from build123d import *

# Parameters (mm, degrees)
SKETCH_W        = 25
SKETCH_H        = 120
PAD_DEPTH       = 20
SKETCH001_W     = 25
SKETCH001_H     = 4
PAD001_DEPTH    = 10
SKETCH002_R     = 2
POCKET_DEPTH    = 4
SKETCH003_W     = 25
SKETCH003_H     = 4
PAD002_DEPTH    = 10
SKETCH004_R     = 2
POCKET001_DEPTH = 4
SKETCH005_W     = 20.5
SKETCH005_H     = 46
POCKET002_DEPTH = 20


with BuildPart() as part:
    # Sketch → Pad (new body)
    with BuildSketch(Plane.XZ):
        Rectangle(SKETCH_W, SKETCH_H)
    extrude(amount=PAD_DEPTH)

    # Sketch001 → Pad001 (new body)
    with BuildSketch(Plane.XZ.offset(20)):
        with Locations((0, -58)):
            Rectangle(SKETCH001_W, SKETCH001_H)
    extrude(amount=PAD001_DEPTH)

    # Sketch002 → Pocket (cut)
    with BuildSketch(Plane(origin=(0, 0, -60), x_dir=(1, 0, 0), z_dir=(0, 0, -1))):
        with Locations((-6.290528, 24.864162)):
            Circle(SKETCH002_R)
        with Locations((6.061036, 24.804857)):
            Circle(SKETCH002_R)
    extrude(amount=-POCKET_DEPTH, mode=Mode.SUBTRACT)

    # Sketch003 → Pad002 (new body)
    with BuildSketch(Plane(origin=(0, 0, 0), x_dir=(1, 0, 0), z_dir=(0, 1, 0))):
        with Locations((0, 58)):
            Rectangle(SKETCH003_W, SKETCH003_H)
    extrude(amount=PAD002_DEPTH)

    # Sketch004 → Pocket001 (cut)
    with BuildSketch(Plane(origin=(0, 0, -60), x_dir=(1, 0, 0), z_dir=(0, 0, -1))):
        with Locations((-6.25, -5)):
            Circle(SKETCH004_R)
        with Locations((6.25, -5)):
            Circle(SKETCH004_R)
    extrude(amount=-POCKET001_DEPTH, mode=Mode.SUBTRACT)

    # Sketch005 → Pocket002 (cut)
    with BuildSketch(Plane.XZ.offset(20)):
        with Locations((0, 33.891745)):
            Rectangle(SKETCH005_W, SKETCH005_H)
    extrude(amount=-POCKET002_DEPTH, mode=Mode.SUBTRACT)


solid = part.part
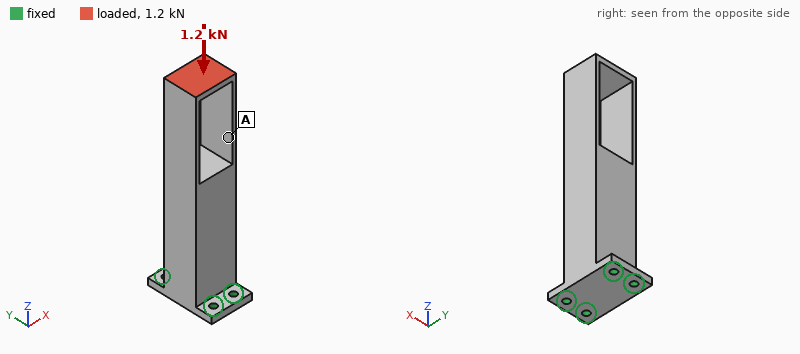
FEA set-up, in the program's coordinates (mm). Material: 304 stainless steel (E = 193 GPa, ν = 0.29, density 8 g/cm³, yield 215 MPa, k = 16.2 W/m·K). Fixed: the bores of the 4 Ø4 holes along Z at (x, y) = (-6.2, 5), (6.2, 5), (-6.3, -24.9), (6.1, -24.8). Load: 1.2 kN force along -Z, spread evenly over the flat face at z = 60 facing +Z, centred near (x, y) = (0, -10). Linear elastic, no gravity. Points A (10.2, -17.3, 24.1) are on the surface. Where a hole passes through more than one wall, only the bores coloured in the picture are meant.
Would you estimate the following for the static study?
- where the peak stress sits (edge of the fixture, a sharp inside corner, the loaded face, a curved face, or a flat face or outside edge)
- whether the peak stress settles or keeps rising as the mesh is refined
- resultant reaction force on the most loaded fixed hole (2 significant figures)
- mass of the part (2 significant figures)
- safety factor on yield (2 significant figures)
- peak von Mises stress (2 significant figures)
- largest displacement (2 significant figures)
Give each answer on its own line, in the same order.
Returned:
a flat face or outside edge
settles
330 N
340 g
2.7
79 MPa
20 µm
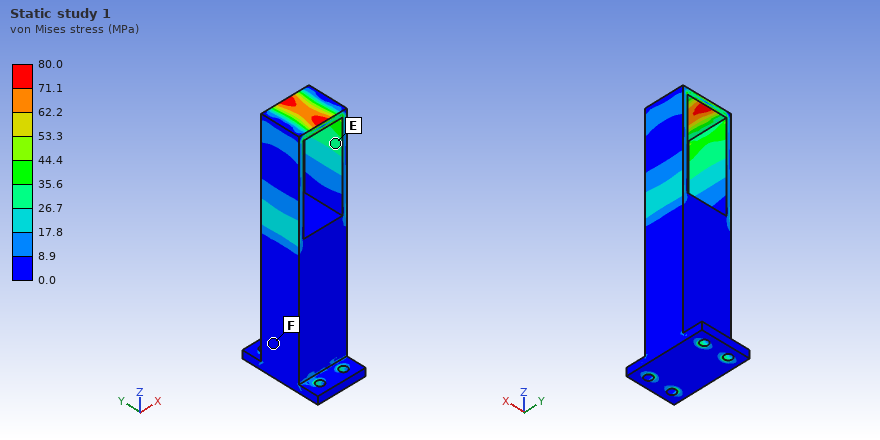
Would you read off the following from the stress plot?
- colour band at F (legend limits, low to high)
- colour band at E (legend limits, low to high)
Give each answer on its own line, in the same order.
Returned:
0.0 to 8.9 MPa
26.7 to 35.6 MPa
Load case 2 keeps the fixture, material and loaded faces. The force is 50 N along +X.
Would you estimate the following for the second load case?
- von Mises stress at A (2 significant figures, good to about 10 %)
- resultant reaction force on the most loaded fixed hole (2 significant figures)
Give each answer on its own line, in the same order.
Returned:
14 MPa
200 N
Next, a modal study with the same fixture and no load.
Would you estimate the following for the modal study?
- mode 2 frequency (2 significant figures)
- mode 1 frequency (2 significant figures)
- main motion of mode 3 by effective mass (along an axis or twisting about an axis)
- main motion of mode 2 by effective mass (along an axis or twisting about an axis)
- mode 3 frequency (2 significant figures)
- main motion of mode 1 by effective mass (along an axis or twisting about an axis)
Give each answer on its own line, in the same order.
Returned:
1400 Hz
750 Hz
along X
along Y
1800 Hz
along X
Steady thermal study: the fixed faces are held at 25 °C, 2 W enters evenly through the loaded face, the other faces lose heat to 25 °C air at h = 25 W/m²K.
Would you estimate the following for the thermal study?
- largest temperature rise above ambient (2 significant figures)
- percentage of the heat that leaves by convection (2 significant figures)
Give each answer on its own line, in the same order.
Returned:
31 K
93 %
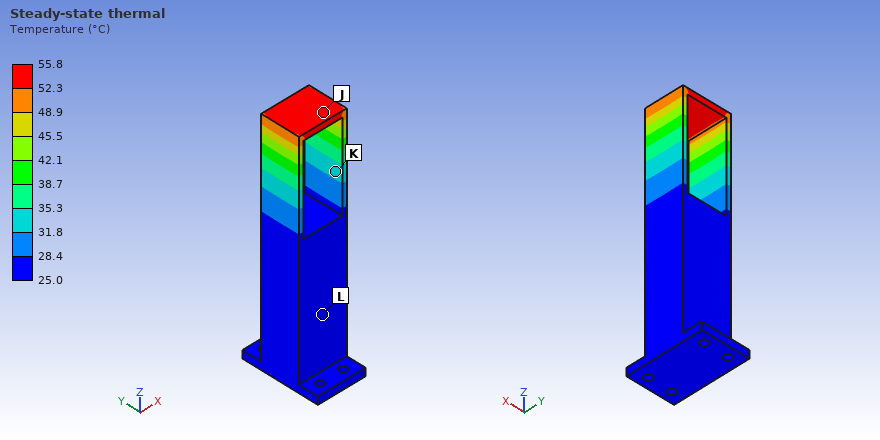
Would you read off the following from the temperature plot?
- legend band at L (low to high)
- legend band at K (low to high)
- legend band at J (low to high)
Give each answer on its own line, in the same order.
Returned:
25.0 to 28.4 °C
31.8 to 35.3 °C
52.3 to 55.8 °C
